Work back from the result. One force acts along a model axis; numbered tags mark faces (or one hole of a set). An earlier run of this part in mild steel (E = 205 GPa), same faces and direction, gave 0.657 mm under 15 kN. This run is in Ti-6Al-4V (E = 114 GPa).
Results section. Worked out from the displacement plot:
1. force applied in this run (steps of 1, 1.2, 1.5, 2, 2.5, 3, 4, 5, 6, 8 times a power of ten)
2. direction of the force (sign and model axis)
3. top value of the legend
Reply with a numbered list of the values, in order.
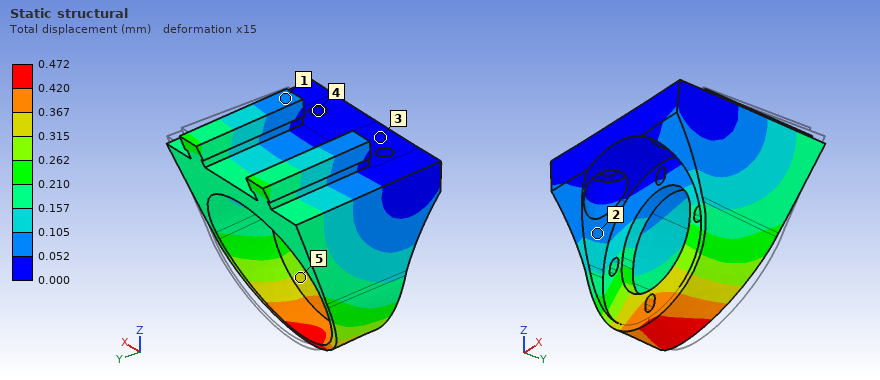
1. 6 kN
2. -Y
3. 0.472 mm
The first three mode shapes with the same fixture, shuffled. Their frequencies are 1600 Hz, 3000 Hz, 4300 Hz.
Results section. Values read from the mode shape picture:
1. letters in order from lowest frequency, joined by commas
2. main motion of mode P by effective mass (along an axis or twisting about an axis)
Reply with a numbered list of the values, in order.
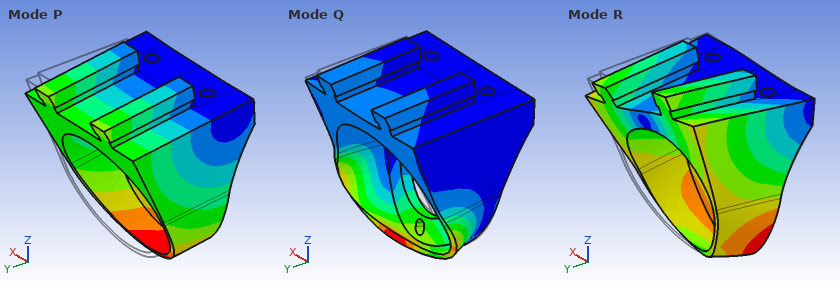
1. P, R, Q
2. along Z
